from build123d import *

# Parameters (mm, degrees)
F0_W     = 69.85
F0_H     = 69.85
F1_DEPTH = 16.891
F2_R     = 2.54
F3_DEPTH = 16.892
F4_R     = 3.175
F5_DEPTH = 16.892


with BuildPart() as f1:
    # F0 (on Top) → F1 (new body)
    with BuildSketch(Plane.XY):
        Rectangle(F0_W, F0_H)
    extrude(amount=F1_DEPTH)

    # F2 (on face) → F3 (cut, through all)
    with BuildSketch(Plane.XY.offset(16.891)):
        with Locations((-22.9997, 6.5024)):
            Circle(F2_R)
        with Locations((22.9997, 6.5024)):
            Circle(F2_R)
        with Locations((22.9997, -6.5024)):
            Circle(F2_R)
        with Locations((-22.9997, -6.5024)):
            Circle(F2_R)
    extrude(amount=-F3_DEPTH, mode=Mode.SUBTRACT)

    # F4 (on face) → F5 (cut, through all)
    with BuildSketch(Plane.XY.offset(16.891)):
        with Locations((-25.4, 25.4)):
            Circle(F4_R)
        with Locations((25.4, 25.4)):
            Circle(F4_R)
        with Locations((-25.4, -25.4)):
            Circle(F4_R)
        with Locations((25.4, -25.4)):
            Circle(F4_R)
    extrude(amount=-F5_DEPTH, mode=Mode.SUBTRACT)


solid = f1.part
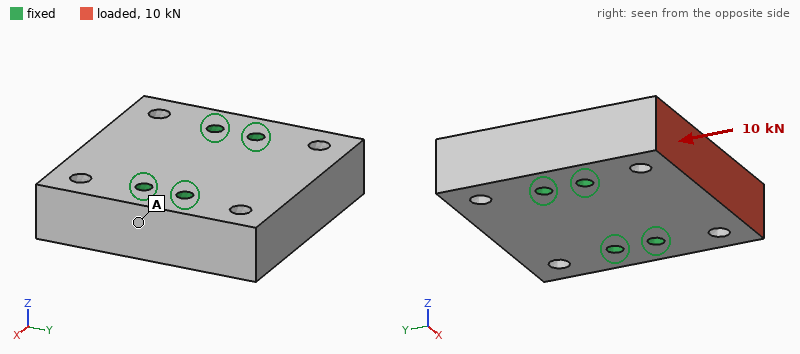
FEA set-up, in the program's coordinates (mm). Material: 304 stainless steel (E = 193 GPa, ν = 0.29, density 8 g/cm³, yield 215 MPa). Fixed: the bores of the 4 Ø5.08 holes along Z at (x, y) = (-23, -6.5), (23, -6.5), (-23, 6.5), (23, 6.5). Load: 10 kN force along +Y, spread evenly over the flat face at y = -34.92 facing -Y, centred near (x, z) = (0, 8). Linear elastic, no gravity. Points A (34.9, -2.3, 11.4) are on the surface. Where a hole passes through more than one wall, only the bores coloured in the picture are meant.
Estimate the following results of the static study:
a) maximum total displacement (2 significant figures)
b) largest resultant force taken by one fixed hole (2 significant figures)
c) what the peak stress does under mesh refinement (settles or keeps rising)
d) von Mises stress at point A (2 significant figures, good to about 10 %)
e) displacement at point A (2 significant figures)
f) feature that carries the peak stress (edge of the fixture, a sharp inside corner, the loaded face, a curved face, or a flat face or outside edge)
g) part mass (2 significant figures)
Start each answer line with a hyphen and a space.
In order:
- 1.9 µm
- 3.5 kN
- keeps rising
- 5.3 MPa
- 0.33 µm
- edge of the fixture
- 630 g
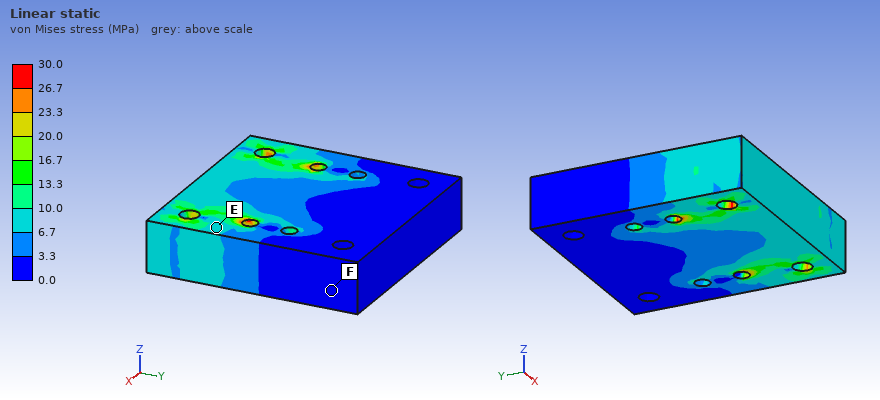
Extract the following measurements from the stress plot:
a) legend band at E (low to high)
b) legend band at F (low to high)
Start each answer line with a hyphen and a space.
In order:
- 6.7 to 10.0 MPa
- 0.0 to 3.3 MPa
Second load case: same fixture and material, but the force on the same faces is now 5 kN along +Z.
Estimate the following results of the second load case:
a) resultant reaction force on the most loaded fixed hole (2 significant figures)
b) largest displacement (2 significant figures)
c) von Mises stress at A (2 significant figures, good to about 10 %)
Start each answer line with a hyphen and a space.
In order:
- 3.5 kN
- 14 µm
- 12 MPa
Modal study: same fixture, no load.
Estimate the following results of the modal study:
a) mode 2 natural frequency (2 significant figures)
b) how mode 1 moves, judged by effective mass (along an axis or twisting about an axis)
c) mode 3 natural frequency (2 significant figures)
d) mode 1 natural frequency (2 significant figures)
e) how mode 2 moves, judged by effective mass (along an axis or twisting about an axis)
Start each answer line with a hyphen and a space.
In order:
- 12 kHz
- twisting about X
- 16 kHz
- 10 kHz
- along Z
